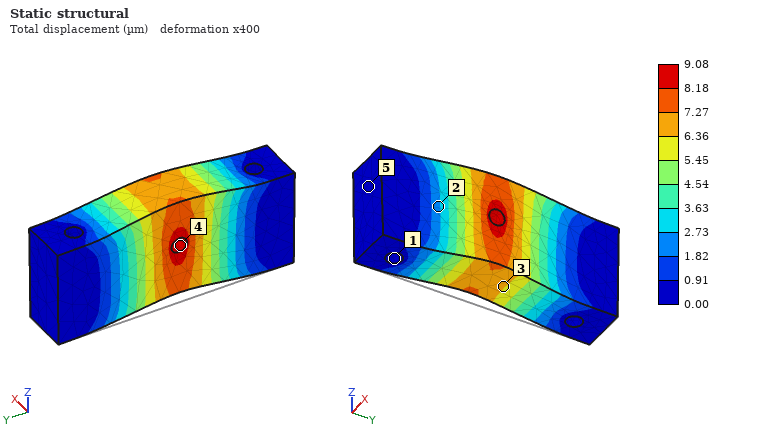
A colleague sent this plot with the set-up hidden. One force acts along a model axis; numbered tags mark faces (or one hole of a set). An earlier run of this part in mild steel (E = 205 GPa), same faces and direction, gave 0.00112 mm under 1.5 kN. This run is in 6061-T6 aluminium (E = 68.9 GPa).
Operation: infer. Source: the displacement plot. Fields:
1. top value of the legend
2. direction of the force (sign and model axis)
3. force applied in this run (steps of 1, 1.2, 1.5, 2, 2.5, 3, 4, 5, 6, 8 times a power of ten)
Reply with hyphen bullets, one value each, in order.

- 9.08 µm
- +Z
- 4 kN
